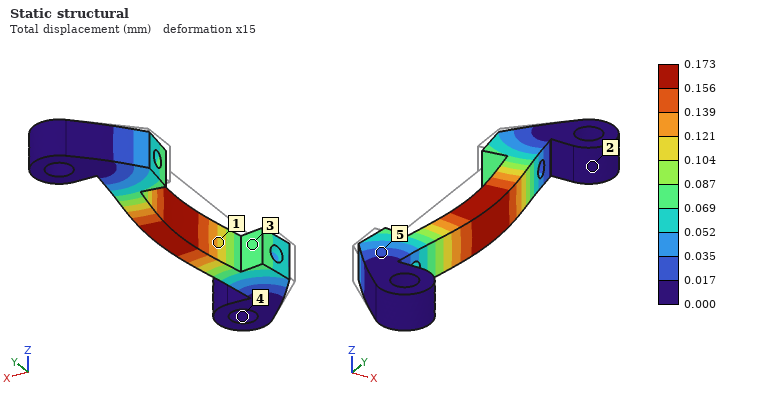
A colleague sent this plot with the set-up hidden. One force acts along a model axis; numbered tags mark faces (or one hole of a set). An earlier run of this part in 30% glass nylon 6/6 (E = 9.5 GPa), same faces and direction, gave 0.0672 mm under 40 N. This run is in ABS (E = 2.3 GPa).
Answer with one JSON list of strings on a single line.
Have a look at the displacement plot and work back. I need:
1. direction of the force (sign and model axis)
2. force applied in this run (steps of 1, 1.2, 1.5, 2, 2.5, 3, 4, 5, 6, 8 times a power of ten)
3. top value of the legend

["+X", "25 N", "0.173 mm"]
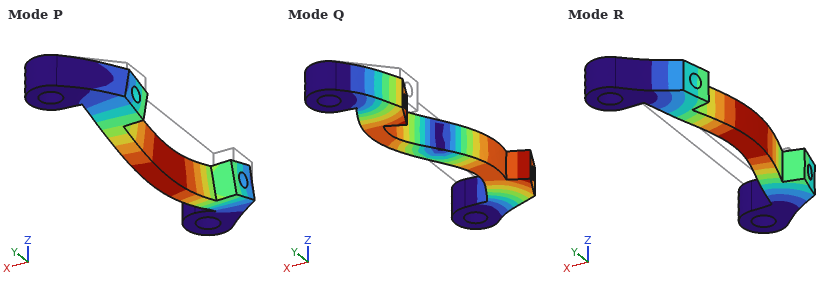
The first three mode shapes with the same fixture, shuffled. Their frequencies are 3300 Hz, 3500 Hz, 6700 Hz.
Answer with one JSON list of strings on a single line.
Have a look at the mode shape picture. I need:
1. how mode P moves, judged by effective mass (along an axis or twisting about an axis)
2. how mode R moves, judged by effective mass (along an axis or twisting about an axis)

["along Z", "along X"]
